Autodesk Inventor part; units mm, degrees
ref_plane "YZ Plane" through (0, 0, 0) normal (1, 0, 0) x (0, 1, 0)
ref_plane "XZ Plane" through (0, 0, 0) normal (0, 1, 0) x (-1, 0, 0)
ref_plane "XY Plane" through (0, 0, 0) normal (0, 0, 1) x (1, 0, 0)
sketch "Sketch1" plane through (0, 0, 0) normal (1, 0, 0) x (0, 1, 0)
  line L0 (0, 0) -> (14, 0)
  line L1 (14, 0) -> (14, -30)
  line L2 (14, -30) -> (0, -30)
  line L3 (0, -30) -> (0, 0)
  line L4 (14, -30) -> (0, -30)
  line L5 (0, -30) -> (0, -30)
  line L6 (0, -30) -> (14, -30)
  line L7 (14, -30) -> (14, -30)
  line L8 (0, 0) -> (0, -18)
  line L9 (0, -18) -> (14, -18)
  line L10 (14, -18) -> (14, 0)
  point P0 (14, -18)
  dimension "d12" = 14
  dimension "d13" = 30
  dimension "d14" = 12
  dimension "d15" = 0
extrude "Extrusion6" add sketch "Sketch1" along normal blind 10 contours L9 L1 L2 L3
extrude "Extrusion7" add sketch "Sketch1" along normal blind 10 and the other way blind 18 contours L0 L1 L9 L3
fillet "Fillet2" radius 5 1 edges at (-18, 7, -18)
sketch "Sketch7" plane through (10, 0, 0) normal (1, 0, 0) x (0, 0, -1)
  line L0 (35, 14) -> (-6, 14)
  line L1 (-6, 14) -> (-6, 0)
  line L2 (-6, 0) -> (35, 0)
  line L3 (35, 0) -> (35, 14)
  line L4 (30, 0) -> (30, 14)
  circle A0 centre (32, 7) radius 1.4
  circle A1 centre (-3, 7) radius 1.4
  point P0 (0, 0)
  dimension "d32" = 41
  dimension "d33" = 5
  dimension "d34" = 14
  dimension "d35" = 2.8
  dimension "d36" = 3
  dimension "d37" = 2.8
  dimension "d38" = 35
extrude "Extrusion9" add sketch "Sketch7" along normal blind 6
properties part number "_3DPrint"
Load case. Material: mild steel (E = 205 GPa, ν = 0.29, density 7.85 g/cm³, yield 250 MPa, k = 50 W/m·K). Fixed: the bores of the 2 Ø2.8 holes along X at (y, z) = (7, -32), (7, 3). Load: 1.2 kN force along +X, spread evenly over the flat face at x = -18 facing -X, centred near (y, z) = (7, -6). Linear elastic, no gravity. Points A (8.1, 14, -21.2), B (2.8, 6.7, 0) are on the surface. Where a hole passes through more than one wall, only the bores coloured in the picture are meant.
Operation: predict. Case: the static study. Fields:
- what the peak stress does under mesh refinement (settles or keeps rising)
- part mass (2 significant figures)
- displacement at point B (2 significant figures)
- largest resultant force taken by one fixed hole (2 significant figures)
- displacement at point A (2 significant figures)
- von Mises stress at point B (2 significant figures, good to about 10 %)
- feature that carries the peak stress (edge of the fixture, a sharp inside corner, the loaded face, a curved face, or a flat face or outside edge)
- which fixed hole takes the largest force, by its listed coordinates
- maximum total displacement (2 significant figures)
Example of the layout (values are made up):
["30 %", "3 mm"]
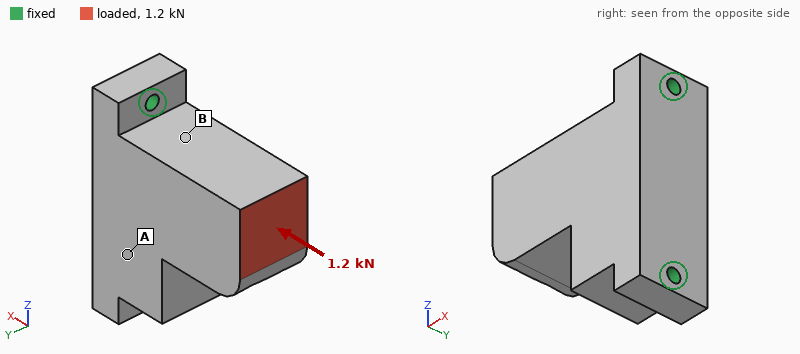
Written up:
["keeps rising", "94 g", "1.8 µm", "940 N", "0.86 µm", "12 MPa", "edge of the fixture", "(7, 3)", "3.0 µm"]
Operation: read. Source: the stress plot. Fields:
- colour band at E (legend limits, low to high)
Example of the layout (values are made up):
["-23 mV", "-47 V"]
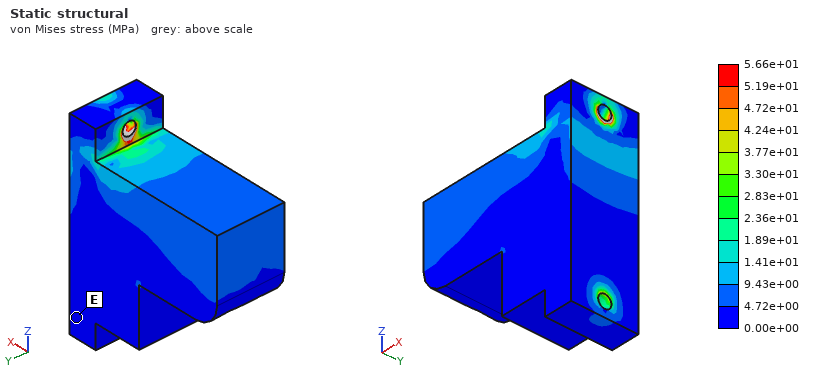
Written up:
["0.00e+00 to 4.72e+00 MPa"]
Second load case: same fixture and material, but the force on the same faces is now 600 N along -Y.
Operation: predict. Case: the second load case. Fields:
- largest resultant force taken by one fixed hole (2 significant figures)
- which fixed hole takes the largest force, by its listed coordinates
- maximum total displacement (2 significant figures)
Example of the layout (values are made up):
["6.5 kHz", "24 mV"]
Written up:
["430 N", "(7, 3)", "36 µm"]
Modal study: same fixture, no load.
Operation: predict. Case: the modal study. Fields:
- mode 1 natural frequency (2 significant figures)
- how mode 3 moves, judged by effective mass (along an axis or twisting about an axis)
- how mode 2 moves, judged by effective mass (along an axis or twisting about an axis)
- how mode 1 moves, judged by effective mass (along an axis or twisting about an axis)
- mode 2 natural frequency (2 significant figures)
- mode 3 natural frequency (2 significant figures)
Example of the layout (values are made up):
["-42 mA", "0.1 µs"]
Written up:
["4600 Hz", "along X", "along Z", "along Y", "13 kHz", "17 kHz"]
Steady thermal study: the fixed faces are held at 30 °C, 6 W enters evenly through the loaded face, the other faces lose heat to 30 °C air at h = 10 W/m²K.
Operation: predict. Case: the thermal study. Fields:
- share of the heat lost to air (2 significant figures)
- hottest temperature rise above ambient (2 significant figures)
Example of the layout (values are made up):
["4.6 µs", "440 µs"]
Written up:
["4.5 %", "19 K"]
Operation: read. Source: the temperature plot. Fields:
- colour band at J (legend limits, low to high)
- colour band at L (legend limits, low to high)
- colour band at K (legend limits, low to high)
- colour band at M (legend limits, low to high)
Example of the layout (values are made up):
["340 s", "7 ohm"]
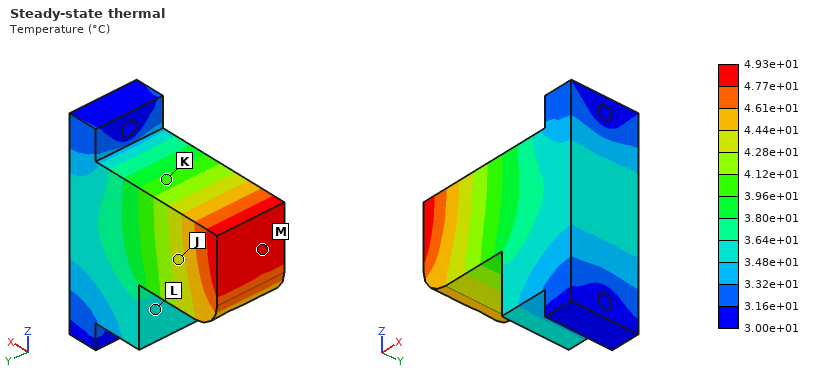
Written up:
["4.28e+01 to 4.44e+01 °C", "3.48e+01 to 3.64e+01 °C", "3.96e+01 to 4.12e+01 °C", "4.77e+01 to 4.93e+01 °C"]
